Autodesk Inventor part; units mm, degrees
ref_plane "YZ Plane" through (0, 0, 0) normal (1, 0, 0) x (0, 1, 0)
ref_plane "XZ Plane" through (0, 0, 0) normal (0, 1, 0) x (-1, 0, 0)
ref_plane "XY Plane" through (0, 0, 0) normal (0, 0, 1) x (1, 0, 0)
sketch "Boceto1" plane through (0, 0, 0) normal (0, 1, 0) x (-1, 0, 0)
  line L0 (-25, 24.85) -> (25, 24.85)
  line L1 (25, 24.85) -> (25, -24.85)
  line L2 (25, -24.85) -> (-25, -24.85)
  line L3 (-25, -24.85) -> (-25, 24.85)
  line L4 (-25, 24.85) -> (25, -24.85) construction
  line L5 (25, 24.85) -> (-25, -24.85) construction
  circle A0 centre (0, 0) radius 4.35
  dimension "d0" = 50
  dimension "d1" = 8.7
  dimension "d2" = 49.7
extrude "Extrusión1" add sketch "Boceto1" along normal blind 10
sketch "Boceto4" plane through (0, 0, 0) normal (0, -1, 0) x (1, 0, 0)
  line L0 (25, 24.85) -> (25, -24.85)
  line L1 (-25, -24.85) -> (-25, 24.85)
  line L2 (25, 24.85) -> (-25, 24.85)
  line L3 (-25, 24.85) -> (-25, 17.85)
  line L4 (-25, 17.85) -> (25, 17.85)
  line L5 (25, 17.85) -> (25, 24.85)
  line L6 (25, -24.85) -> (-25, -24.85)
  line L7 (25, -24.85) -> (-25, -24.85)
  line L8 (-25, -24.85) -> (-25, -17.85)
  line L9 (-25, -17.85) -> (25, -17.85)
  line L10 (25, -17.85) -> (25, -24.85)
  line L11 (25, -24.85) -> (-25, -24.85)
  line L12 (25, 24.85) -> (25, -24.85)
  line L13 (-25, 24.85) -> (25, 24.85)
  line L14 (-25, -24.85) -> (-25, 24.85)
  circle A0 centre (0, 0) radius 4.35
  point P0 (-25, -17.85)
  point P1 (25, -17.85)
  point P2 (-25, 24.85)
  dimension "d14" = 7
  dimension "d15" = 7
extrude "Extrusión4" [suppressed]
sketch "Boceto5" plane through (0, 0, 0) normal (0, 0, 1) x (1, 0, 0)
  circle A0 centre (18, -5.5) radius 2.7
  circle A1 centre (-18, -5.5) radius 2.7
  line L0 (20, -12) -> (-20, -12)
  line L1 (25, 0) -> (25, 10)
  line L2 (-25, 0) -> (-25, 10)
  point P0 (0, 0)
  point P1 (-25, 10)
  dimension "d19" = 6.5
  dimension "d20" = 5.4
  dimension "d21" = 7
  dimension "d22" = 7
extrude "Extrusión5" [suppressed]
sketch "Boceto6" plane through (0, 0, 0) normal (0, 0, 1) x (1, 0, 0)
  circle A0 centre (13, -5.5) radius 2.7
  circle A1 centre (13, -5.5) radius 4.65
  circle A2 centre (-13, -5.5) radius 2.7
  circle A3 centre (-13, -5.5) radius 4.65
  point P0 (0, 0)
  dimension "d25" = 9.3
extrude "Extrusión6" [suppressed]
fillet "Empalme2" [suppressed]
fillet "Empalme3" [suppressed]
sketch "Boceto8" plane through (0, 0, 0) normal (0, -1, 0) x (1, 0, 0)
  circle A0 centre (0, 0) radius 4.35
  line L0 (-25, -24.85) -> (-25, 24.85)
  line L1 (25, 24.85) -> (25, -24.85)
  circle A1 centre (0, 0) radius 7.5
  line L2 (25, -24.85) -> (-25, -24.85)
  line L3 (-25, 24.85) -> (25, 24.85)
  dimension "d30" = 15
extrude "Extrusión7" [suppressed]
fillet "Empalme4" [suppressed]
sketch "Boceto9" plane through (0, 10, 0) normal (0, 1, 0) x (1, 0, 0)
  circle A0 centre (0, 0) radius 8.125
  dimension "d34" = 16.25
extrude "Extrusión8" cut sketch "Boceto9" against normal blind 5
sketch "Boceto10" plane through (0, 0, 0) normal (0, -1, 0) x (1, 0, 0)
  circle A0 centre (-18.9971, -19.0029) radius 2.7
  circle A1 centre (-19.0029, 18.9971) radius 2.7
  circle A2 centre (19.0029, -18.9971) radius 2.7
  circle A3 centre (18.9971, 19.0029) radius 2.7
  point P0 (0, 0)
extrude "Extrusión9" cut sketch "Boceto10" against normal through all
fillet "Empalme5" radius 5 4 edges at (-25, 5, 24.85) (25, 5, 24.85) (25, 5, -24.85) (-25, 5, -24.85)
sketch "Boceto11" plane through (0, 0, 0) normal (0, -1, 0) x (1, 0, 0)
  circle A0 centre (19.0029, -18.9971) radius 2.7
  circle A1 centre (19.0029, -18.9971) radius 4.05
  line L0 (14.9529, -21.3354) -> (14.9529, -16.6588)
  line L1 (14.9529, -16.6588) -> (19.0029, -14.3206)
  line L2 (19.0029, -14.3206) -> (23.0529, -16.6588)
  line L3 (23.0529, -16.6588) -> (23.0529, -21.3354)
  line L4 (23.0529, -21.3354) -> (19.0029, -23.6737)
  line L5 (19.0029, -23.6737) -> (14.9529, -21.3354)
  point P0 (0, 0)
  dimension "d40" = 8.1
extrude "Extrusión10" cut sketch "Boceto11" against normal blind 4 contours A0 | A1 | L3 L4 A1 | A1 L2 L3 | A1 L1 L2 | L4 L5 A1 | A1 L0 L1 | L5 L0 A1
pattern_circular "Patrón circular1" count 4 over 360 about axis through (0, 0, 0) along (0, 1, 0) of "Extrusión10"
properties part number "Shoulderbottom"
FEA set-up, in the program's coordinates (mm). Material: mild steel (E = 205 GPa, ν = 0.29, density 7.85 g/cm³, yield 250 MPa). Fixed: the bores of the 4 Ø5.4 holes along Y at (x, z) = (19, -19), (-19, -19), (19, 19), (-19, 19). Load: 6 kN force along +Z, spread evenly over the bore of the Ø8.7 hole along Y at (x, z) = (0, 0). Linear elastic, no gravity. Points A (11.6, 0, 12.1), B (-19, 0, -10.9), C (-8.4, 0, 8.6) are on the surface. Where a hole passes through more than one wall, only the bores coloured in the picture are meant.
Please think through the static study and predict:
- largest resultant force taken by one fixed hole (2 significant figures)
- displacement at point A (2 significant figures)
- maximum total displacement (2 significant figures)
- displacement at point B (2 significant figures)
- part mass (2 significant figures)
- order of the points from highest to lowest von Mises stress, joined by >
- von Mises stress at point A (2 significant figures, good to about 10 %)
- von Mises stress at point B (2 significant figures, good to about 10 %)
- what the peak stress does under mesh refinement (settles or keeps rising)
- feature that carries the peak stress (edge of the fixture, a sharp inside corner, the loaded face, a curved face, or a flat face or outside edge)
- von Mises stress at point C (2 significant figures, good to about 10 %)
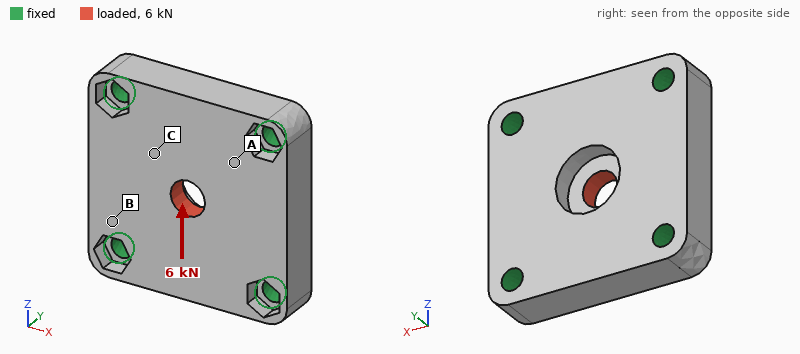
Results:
1.7 kN
1.2 µm
3.4 µm
0.60 µm
170 g
C > A > B
14 MPa
7.2 MPa
keeps rising
a sharp inside corner
22 MPa
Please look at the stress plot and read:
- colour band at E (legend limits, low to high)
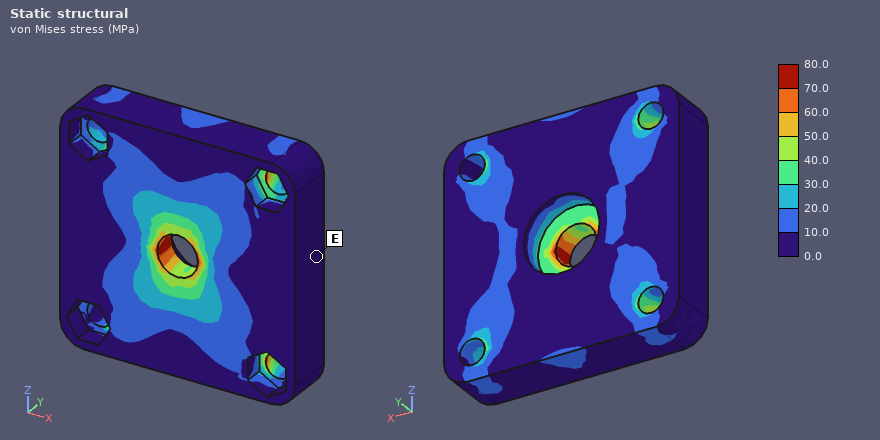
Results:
0.0 to 10.0 MPa
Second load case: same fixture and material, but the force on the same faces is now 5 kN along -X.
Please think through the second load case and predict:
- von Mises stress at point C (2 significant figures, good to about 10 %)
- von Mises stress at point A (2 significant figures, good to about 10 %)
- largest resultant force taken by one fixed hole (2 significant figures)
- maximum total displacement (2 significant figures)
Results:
18 MPa
12 MPa
1.4 kN
2.8 µm
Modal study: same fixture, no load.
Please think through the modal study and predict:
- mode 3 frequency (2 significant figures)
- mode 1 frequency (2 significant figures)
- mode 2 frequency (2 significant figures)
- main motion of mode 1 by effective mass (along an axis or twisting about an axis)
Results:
26 kHz
18 kHz
26 kHz
along Y
